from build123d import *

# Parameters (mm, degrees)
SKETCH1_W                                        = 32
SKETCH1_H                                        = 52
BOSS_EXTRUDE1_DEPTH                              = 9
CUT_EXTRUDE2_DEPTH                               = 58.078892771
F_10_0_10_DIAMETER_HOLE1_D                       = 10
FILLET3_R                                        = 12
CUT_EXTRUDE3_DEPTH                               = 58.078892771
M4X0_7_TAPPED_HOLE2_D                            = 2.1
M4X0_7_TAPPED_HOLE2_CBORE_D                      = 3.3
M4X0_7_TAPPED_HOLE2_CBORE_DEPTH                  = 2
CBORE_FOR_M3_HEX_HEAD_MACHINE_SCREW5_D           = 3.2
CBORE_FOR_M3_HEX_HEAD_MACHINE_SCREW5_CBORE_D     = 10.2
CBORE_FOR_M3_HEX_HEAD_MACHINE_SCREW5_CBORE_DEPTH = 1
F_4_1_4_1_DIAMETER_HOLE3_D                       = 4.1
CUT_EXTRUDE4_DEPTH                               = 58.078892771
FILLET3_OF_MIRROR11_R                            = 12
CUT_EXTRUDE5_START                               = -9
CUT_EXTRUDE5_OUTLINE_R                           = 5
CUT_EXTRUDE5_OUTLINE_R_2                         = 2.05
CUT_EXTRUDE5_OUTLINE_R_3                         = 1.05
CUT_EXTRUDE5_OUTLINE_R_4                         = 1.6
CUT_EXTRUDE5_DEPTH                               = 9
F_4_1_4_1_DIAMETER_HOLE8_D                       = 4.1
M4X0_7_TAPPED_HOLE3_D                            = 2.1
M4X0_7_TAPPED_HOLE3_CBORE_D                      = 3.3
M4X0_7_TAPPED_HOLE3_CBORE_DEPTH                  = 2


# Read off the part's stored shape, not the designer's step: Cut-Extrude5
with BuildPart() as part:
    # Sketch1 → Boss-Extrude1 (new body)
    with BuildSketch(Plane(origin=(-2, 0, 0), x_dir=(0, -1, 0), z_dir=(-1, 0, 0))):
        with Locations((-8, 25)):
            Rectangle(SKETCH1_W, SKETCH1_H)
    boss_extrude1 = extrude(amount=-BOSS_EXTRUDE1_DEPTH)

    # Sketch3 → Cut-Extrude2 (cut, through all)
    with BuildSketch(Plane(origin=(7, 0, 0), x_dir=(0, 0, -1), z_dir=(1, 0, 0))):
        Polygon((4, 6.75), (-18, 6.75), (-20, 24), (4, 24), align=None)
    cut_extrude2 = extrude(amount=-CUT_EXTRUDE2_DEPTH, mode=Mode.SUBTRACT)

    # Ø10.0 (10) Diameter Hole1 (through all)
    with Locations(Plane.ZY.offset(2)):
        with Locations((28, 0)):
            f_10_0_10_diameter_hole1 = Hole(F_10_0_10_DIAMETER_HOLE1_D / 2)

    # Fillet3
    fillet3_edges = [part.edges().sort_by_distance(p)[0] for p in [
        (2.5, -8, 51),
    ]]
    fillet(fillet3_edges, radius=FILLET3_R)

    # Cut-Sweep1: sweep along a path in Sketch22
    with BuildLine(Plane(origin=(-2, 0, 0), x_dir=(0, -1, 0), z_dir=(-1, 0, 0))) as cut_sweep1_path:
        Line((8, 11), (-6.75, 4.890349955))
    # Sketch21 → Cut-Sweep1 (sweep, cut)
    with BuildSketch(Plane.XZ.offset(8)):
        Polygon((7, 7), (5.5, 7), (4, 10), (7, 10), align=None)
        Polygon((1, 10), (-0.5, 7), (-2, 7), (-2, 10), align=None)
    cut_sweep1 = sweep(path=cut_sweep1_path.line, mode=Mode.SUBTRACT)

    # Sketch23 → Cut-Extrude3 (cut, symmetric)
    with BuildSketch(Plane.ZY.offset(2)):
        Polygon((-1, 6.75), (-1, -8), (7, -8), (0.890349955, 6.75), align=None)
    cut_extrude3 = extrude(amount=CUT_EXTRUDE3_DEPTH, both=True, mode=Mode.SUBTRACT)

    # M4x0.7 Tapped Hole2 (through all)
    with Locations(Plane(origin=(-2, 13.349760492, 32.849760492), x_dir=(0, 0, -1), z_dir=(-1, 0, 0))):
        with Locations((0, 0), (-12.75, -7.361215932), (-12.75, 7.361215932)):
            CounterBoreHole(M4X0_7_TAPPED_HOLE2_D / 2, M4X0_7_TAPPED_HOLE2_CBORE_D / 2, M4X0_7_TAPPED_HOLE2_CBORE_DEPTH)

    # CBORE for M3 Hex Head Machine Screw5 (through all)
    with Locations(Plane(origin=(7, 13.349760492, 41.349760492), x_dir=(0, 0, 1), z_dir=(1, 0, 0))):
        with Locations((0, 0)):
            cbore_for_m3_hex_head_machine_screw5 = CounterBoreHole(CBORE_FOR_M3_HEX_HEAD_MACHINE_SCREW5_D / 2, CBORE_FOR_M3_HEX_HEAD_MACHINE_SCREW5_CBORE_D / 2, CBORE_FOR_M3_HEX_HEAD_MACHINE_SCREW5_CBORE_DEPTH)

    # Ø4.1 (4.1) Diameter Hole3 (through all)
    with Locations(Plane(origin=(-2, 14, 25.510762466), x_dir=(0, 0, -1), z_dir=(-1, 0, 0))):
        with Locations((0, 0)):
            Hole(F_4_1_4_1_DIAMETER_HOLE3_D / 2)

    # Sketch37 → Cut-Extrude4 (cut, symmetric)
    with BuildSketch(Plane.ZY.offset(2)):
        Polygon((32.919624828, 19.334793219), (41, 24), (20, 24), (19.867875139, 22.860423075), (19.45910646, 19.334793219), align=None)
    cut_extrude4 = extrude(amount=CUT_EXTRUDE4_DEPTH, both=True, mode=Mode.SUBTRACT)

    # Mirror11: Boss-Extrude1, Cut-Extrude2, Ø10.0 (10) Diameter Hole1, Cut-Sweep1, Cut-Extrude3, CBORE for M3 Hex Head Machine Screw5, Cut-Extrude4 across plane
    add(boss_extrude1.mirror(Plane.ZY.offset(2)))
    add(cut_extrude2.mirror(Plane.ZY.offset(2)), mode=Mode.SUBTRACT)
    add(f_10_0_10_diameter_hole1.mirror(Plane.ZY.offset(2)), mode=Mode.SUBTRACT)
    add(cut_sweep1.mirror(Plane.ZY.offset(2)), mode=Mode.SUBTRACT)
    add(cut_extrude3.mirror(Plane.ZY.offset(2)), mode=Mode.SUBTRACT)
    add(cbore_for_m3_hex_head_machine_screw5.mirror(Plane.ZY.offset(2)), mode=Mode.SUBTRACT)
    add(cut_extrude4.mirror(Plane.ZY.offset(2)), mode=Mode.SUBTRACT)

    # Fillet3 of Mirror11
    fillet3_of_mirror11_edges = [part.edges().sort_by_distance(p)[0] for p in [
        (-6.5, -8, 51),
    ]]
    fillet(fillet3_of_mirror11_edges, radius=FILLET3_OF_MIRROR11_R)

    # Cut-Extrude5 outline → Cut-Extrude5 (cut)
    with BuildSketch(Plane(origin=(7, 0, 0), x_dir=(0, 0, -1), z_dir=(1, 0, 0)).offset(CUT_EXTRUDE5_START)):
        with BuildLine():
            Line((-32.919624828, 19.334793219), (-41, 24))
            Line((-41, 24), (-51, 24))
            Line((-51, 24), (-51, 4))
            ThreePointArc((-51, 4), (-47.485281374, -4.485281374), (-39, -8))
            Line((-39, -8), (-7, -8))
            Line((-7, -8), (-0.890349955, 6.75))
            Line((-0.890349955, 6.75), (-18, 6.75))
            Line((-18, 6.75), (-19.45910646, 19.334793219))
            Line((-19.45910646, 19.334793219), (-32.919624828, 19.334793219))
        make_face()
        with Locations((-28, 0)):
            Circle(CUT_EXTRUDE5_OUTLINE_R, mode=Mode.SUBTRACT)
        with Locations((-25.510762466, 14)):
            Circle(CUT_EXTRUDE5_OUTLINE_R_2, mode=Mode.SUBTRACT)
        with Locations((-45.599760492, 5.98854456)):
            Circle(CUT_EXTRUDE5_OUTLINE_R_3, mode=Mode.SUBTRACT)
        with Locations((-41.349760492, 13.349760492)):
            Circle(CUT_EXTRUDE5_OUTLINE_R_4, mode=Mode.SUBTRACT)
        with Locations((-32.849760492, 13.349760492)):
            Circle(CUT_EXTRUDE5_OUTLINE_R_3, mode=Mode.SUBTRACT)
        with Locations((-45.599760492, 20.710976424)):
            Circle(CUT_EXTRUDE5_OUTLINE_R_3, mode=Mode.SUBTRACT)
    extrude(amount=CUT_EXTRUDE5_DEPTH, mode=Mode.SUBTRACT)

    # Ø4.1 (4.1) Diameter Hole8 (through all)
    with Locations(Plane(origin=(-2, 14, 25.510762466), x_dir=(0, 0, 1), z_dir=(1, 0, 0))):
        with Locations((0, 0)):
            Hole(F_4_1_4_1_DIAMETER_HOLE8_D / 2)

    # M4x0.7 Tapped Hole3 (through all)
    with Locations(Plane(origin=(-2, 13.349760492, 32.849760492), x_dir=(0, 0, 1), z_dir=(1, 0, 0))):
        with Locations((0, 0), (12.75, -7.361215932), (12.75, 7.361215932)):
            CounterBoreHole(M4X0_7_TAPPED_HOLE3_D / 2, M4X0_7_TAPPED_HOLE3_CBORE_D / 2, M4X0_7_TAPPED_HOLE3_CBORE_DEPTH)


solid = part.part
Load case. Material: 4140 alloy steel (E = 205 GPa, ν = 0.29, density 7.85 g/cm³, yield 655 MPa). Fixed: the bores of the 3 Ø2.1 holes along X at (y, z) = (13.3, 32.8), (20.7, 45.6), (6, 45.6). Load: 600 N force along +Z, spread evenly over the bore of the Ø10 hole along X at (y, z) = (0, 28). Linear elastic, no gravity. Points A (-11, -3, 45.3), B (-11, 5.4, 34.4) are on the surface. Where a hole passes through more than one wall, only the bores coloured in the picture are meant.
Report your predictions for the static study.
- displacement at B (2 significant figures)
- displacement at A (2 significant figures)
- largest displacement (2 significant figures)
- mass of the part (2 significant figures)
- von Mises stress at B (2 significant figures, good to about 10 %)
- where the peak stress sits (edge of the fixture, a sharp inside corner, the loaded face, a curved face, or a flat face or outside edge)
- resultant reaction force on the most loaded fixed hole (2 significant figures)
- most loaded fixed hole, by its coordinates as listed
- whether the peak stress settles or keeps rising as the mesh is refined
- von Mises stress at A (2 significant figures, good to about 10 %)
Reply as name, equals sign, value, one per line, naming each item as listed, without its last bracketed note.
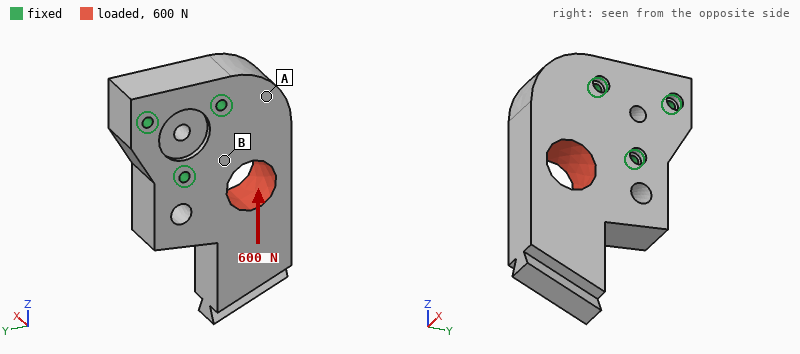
displacement at B = 0.34 µm
displacement at A = 0.57 µm
largest displacement = 1.9 µm
mass of the part = 70 g
von Mises stress at B = 7.7 MPa
where the peak stress sits = edge of the fixture
resultant reaction force on the most loaded fixed hole = 520 N
most loaded fixed hole, by its coordinates as listed = (6, 45.6)
whether the peak stress settles or keeps rising as the mesh is refined = keeps rising
von Mises stress at A = 2.7 MPa
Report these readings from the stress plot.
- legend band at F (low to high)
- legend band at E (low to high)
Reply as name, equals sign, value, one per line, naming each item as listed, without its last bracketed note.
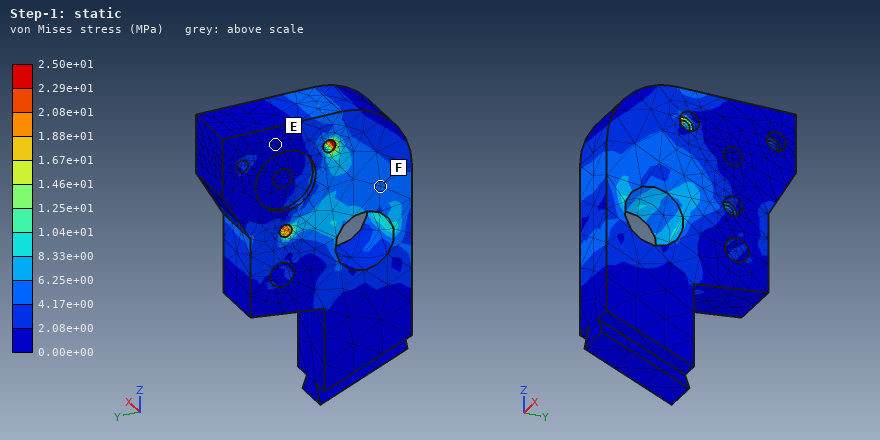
legend band at F = 4.17e+00 to 6.25e+00 MPa
legend band at E = 0.00e+00 to 2.08e+00 MPa
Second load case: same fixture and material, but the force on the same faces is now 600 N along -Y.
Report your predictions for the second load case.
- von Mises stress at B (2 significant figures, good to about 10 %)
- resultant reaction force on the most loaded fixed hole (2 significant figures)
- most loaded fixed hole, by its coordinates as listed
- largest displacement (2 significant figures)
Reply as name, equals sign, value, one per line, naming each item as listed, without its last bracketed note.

von Mises stress at B = 9.0 MPa
resultant reaction force on the most loaded fixed hole = 620 N
most loaded fixed hole, by its coordinates as listed = (13.3, 32.8)
largest displacement = 1.6 µm
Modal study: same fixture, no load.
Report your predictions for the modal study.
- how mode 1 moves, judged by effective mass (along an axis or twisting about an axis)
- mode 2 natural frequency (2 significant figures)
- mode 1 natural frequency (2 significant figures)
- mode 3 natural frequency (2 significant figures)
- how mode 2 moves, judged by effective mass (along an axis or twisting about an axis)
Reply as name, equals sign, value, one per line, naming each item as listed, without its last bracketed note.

how mode 1 moves, judged by effective mass = along X
mode 2 natural frequency = 12 kHz
mode 1 natural frequency = 5900 Hz
mode 3 natural frequency = 16 kHz
how mode 2 moves, judged by effective mass = along Y
